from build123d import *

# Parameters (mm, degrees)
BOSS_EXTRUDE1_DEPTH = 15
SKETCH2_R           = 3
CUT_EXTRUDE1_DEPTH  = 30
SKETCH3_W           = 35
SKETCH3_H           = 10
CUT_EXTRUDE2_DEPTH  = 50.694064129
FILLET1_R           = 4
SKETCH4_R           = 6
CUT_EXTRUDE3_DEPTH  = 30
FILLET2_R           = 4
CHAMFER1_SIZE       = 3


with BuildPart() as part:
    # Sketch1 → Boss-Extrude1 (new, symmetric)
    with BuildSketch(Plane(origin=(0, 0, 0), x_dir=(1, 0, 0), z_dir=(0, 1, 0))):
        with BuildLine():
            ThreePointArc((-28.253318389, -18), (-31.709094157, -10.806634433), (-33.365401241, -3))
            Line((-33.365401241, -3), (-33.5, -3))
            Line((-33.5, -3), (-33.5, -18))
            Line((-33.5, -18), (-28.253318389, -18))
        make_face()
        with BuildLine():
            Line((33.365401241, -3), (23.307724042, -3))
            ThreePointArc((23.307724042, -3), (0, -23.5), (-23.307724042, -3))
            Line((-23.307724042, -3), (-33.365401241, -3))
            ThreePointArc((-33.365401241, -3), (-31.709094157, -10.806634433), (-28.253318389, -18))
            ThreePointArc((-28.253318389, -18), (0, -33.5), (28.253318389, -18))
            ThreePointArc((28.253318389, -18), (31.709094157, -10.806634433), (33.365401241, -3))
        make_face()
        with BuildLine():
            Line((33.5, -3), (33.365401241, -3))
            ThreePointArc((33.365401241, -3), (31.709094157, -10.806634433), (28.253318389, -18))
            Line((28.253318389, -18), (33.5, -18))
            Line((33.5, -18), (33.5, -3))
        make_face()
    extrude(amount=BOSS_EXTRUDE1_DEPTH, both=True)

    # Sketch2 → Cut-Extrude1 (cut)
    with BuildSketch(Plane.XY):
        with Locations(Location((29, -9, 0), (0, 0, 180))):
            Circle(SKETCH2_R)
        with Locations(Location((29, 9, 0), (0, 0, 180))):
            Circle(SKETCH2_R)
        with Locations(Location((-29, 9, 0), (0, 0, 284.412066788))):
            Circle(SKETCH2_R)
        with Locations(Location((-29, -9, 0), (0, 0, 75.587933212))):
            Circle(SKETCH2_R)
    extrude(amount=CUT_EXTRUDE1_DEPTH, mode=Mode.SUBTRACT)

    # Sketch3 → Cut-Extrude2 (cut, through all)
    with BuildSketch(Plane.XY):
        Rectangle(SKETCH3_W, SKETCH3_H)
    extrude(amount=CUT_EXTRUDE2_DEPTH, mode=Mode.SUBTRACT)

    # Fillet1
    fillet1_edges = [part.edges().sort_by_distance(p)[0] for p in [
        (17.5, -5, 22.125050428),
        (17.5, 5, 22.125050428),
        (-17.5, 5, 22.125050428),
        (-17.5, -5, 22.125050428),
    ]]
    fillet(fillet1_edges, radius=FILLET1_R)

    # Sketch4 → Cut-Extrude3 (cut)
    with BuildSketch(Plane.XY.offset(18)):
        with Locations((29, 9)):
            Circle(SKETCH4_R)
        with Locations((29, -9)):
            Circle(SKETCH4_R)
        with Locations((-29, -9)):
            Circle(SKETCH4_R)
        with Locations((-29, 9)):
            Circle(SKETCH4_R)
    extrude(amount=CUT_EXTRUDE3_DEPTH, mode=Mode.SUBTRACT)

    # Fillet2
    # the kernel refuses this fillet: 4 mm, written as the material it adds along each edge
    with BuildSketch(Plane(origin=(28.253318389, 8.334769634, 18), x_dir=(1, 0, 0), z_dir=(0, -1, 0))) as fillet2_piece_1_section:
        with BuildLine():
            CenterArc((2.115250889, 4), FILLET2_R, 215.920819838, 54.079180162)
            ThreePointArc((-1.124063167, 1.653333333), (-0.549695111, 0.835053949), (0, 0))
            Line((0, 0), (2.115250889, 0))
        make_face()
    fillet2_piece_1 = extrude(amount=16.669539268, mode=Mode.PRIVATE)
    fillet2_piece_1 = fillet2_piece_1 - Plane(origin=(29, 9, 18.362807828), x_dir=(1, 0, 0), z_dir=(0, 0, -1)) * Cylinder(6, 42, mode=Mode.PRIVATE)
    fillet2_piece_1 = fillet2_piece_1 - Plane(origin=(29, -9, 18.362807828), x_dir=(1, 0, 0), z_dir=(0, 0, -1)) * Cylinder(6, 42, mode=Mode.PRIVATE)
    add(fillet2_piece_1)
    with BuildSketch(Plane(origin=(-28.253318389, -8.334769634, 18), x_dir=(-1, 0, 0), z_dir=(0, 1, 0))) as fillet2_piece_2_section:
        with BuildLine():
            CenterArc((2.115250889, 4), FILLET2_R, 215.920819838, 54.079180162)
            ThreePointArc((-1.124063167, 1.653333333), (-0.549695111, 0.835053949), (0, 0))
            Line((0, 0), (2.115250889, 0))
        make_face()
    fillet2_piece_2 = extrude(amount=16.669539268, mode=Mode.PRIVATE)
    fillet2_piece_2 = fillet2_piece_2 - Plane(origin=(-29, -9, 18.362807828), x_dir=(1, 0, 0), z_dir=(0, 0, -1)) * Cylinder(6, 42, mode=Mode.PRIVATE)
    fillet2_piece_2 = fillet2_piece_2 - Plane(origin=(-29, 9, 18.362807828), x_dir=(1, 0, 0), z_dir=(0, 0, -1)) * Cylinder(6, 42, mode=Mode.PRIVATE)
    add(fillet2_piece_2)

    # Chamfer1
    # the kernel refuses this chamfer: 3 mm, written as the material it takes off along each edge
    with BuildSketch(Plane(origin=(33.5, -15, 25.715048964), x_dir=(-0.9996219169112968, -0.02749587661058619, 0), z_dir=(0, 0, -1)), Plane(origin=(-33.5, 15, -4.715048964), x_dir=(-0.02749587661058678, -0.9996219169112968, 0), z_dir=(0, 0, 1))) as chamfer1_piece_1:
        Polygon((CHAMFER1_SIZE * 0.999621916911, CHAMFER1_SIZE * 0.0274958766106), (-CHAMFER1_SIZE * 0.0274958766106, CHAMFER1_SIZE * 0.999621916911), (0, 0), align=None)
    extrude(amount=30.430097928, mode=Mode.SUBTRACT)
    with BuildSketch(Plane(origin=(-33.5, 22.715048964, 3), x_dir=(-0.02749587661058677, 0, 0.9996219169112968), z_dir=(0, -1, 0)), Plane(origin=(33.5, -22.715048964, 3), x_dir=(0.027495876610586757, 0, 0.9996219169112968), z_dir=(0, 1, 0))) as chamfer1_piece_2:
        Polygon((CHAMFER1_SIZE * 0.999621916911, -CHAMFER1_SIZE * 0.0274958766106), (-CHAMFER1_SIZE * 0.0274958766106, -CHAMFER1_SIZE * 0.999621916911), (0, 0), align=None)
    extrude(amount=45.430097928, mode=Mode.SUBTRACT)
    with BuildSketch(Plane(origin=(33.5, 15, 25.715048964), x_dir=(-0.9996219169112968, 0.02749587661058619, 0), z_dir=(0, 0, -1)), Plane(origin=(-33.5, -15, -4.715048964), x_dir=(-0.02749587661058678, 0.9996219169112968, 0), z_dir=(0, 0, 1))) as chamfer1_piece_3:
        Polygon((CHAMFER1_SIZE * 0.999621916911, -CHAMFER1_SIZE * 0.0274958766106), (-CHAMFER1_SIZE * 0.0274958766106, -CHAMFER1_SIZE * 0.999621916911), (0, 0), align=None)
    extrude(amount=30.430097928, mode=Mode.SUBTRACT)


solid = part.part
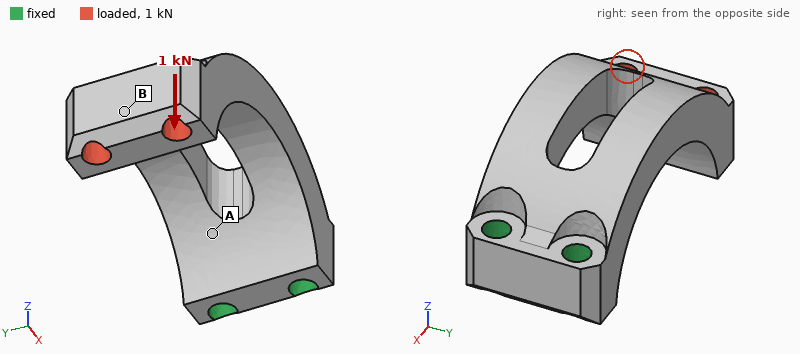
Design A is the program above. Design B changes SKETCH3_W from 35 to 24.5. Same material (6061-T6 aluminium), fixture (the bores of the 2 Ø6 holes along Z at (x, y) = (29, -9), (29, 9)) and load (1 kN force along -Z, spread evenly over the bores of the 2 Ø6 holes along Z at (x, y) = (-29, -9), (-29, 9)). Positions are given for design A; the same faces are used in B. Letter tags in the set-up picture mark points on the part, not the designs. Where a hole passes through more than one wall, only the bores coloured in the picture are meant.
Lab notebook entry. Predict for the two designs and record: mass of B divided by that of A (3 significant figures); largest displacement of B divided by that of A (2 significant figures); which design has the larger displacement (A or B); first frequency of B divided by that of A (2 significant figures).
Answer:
1.06
0.92
A
1.0
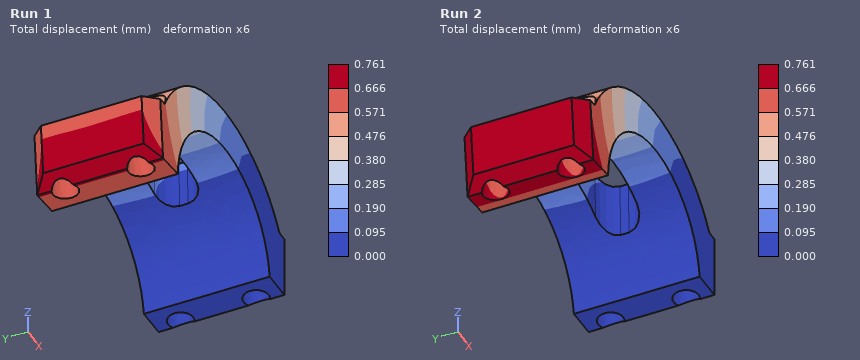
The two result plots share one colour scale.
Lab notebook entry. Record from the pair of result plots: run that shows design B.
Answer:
Run 1
